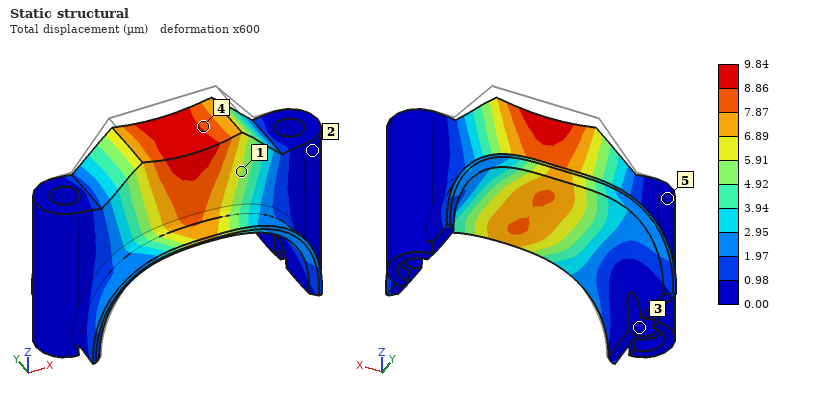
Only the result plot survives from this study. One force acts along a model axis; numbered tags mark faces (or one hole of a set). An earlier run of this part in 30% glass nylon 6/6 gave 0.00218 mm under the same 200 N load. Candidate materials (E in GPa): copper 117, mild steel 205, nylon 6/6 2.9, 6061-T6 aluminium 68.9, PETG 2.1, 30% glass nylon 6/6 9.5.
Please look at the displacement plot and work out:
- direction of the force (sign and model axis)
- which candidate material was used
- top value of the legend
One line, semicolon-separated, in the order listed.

-Z; PETG; 9.84 µm
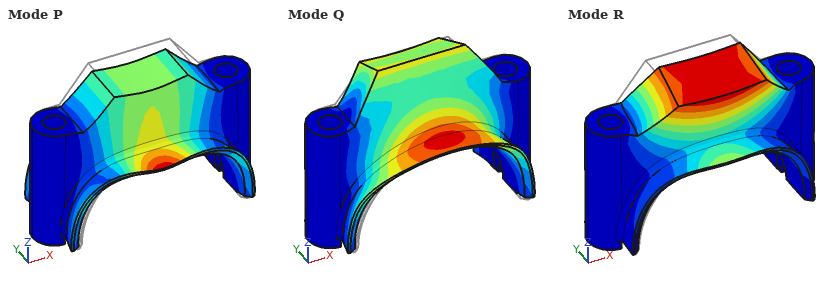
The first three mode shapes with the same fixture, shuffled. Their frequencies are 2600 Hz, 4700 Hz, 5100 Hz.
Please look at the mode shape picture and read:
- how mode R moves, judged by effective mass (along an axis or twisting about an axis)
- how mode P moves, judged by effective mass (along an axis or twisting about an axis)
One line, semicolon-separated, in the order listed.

along Y; along Z
